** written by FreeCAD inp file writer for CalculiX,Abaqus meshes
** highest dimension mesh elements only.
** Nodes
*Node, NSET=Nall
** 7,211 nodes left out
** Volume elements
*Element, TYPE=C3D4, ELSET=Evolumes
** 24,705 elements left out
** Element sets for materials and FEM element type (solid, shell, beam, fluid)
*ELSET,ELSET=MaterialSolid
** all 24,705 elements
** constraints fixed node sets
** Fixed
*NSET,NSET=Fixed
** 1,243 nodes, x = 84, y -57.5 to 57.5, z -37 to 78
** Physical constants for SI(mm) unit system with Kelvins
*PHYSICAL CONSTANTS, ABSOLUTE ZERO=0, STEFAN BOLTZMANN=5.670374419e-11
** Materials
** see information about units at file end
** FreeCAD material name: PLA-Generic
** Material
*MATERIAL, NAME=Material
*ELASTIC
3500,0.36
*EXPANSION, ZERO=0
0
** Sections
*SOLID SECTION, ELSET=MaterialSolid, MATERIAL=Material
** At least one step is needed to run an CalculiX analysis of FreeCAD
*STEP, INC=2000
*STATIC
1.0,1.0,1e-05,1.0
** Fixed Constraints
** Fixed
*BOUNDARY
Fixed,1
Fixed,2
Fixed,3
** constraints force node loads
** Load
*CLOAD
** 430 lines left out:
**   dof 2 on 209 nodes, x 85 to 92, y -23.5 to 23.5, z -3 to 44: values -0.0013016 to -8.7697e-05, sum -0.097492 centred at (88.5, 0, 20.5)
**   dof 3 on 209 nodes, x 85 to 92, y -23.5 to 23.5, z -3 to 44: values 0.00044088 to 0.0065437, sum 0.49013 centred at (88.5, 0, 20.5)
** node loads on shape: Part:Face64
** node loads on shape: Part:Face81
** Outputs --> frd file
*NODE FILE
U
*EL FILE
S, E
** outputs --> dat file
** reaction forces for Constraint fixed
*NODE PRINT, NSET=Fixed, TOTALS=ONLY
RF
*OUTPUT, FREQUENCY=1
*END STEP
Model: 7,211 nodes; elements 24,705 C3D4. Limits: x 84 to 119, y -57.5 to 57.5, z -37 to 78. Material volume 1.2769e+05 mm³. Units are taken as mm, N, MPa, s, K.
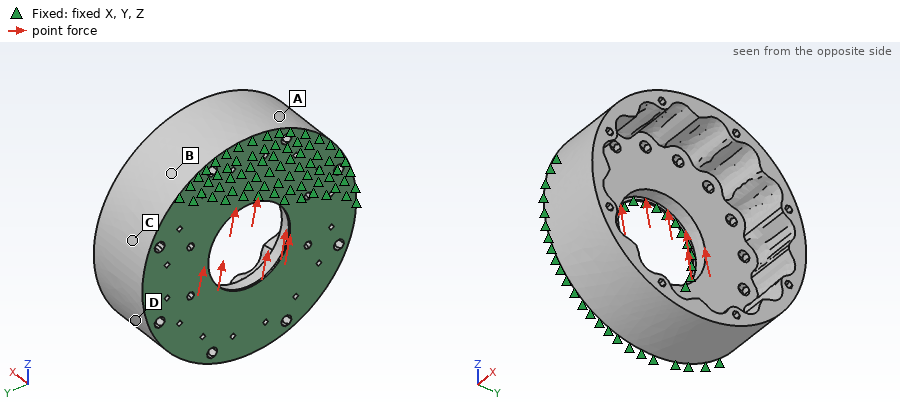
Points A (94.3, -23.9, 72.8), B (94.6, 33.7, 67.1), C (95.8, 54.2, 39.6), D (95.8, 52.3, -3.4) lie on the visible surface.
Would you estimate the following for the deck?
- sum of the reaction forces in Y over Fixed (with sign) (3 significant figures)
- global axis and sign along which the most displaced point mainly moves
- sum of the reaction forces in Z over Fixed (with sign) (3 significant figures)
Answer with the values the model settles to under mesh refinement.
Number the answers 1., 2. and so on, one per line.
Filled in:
1. 0.0975 N
2. +Z
3. -0.490 N
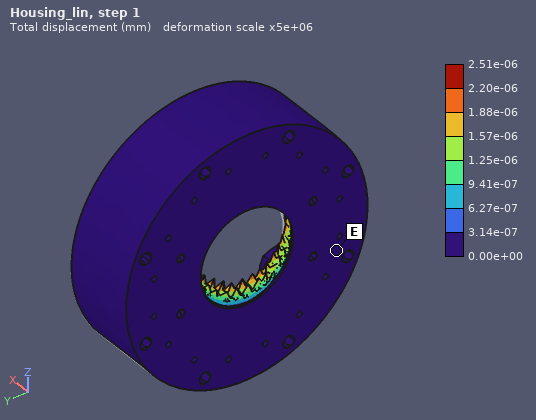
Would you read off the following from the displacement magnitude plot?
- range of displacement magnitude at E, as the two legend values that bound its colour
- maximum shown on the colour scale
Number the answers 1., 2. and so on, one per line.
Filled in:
1. 0.00e+00 to 3.14e-07 mm
2. 2.51e-06 mm
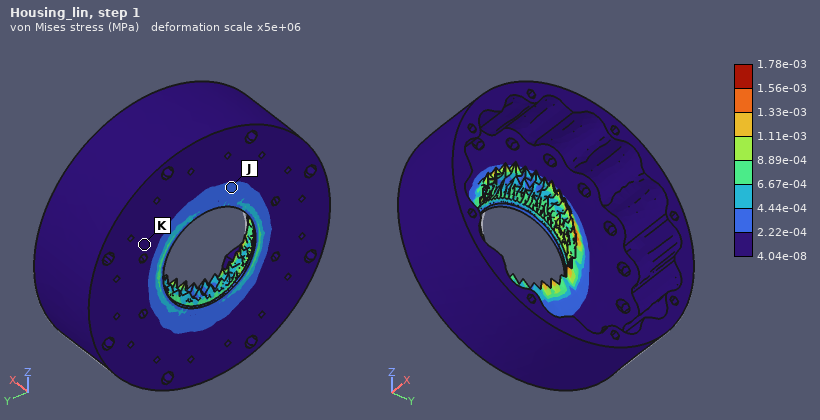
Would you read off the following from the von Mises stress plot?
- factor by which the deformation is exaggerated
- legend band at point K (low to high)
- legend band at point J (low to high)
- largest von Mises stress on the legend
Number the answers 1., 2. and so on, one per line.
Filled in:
1. 5e+06
2. 4.04e-08 to 2.22e-04 MPa
3. 2.22e-04 to 4.44e-04 MPa
4. 1.78e-03 MPa
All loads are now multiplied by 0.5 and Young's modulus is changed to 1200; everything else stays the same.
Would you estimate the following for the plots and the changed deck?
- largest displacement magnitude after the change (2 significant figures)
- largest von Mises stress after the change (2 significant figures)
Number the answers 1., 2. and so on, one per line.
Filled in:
1. 3.7e-06 mm
2. 8.9e-04 MPa
